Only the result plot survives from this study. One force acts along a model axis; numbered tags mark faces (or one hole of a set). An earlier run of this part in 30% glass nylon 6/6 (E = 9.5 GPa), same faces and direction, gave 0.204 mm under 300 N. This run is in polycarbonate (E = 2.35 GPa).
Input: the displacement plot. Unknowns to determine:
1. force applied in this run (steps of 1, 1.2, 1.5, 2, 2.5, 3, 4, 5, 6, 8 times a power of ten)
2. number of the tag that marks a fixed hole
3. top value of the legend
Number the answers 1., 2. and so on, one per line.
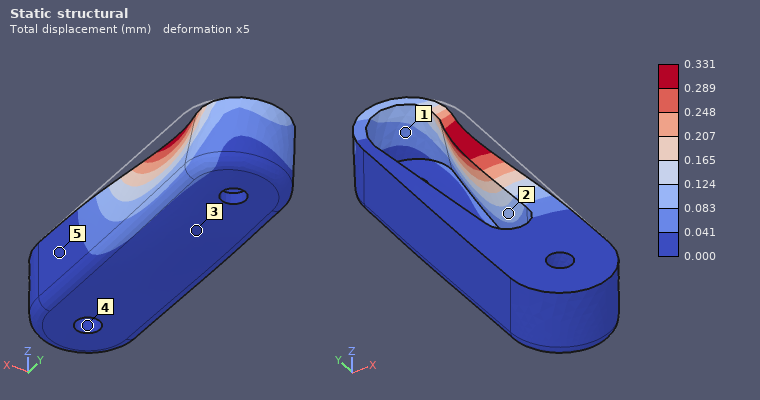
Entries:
1. 120 N
2. 4
3. 0.331 mm
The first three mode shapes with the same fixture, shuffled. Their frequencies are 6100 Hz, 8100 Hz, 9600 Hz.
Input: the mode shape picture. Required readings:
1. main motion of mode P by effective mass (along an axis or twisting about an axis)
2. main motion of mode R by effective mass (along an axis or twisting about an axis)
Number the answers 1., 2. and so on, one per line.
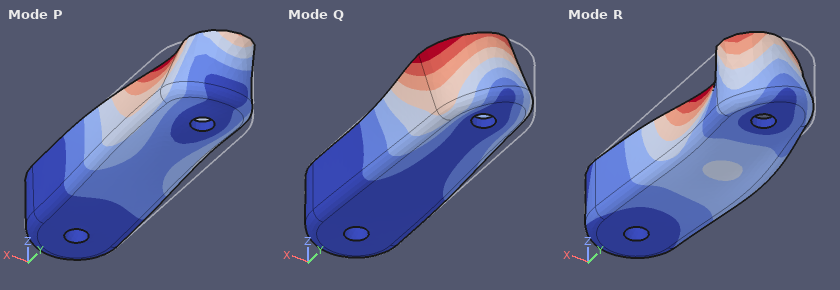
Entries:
1. along Z
2. along X
